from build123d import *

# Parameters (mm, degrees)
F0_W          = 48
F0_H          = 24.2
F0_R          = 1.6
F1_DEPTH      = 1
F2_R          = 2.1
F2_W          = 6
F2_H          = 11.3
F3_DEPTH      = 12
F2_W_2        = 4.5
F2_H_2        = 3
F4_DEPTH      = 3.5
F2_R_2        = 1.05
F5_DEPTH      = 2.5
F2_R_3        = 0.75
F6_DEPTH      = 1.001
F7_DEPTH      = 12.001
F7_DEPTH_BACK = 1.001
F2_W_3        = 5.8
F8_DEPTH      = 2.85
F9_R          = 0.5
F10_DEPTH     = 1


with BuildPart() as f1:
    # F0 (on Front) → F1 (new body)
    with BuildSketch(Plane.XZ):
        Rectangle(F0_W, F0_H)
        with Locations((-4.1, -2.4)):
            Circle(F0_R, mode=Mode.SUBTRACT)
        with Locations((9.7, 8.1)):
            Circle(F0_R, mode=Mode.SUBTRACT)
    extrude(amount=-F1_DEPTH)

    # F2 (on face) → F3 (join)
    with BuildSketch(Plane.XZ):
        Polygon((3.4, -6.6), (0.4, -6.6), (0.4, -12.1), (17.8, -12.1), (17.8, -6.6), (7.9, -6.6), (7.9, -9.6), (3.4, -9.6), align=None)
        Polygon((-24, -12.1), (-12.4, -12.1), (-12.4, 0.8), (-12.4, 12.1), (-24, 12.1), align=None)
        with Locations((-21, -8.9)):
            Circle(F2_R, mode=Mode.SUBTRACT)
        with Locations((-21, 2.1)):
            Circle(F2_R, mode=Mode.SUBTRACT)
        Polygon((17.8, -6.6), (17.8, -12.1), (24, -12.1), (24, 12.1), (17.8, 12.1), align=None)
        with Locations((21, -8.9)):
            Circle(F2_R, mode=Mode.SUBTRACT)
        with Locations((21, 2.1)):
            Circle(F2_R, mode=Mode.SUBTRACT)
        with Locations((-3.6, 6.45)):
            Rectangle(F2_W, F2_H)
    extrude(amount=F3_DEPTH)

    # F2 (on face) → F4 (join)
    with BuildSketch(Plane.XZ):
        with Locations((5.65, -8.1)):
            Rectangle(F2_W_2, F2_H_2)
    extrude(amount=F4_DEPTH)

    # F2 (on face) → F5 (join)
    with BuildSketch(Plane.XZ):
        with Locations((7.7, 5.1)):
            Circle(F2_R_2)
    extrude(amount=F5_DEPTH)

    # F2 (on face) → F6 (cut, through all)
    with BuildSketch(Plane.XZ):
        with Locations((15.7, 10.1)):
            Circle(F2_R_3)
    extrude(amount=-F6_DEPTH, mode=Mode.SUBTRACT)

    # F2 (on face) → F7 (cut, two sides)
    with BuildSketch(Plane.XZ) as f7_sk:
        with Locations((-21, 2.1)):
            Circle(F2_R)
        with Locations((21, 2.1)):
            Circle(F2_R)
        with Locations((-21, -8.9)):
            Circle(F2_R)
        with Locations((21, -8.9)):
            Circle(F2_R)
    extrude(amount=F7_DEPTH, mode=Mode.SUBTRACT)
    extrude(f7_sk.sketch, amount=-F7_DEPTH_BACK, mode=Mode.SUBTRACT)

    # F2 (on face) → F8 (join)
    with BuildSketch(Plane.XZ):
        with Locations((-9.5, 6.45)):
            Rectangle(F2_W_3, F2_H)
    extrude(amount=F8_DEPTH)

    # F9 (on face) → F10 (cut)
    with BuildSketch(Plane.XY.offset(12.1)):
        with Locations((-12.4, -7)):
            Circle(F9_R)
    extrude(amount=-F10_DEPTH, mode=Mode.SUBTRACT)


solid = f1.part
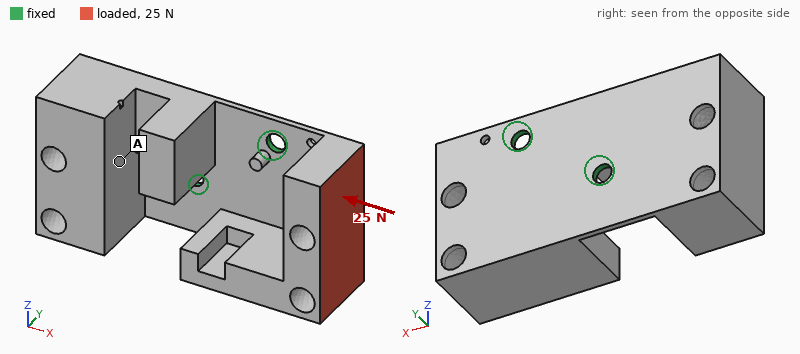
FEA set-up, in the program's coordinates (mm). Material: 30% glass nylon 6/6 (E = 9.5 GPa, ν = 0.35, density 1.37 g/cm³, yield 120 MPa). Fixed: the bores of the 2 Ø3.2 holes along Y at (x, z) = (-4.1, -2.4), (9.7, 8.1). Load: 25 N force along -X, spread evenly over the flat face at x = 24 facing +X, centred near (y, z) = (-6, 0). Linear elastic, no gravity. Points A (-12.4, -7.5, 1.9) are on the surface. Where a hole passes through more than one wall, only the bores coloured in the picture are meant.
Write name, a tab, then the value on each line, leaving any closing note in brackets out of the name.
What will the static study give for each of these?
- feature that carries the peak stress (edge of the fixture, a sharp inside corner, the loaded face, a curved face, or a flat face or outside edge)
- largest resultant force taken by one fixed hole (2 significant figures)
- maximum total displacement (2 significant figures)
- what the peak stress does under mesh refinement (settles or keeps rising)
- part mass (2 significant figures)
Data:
feature that carries the peak stress	edge of the fixture
largest resultant force taken by one fixed hole	15 N
maximum total displacement	0.59 mm
what the peak stress does under mesh refinement	keeps rising
part mass	10 g
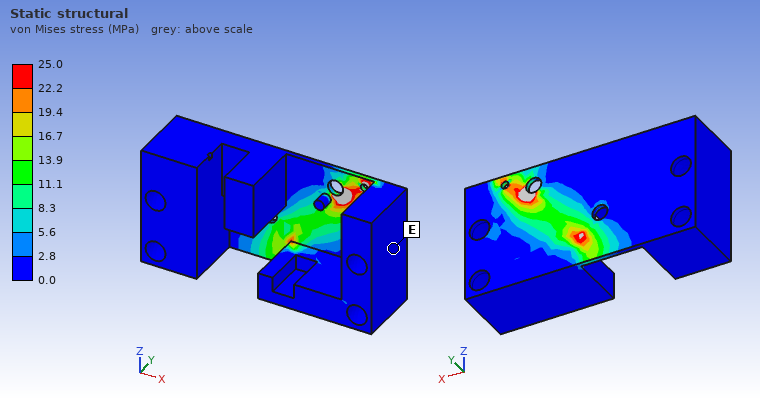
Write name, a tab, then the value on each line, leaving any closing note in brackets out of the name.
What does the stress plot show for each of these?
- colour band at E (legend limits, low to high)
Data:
colour band at E	0.0 to 2.8 MPa
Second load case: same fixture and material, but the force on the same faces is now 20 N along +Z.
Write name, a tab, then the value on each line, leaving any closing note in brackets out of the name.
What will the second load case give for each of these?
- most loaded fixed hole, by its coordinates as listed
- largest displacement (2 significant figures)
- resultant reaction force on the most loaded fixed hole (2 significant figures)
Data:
most loaded fixed hole, by its coordinates as listed	(9.7, 8.1)
largest displacement	0.53 mm
resultant reaction force on the most loaded fixed hole	30 N
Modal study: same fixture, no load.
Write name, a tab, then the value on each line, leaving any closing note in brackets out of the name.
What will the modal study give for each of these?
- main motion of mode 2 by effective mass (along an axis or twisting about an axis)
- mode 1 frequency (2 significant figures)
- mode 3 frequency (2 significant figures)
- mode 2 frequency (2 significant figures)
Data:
main motion of mode 2 by effective mass	along Y
mode 1 frequency	410 Hz
mode 3 frequency	930 Hz
mode 2 frequency	520 Hz
